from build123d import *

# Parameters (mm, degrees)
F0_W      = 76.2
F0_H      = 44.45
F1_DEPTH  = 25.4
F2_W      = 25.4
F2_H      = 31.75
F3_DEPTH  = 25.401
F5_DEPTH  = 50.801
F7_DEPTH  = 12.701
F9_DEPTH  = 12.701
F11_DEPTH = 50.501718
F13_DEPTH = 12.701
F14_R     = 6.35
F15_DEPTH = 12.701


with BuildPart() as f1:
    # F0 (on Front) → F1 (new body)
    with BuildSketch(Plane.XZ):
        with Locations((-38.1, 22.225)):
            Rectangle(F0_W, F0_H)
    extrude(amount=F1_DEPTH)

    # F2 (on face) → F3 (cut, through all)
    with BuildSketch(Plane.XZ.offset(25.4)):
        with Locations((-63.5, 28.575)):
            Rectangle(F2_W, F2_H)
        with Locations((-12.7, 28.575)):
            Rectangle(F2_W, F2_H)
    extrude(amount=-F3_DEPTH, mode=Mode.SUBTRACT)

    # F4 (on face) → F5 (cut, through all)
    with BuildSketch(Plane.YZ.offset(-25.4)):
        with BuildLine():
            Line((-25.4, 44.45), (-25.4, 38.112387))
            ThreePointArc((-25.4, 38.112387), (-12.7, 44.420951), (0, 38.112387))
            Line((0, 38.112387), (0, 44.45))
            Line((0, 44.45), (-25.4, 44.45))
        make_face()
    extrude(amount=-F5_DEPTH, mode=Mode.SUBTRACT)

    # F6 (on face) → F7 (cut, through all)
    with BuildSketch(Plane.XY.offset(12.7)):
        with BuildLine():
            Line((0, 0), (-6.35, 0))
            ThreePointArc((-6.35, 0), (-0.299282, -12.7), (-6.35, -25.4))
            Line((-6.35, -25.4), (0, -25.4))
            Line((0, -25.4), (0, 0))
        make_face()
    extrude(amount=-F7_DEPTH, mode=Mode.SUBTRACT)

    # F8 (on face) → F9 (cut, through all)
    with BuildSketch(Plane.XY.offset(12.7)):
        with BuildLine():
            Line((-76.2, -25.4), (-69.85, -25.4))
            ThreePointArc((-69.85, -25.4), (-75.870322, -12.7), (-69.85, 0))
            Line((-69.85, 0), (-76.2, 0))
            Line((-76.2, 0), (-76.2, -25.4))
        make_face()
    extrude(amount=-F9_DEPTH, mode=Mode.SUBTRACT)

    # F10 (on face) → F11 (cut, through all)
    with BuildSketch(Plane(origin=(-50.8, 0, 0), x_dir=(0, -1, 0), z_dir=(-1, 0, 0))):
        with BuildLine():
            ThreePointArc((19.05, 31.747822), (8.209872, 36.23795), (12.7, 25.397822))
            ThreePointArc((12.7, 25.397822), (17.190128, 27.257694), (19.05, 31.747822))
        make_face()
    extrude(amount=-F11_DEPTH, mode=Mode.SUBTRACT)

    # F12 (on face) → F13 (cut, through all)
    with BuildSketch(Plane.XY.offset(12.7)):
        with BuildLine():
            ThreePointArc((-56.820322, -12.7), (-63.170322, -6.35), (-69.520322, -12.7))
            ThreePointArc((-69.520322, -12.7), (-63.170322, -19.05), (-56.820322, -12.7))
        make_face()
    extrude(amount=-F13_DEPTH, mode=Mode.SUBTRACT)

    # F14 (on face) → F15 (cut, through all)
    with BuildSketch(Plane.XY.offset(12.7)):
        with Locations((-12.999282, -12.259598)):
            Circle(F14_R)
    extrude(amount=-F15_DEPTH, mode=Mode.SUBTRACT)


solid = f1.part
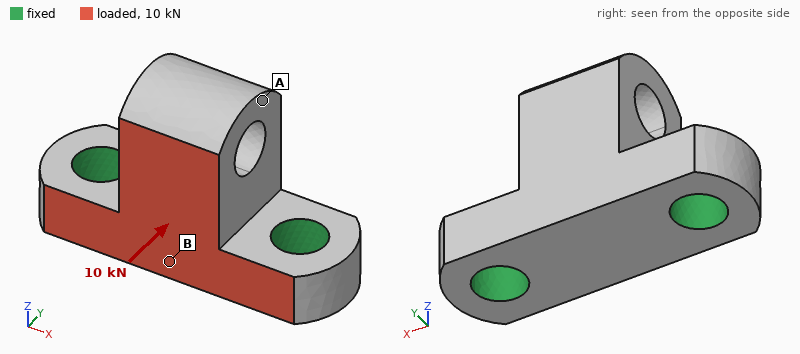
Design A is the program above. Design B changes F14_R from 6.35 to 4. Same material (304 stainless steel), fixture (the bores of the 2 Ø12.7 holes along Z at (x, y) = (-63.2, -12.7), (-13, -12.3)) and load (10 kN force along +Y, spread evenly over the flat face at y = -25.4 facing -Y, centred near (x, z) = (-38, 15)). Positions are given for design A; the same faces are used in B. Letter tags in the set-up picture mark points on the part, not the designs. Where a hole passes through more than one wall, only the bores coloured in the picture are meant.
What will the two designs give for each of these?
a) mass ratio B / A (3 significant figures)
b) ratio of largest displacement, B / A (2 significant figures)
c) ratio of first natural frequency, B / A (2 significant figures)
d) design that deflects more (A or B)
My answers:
1.03
1.1
0.94
B
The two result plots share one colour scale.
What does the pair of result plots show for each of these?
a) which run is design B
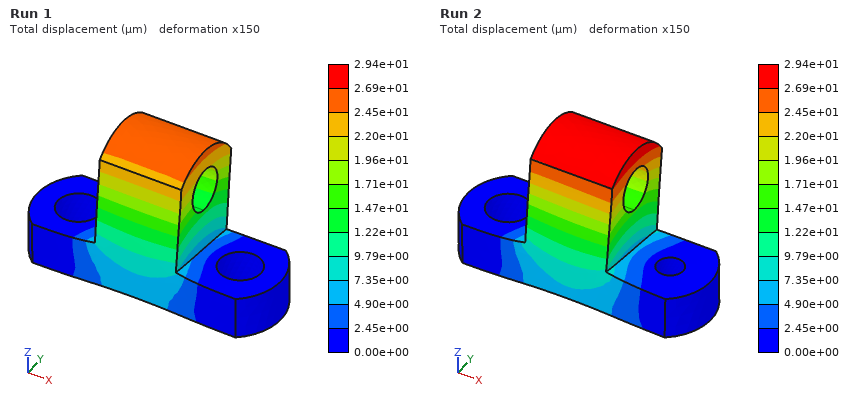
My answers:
Run 2
